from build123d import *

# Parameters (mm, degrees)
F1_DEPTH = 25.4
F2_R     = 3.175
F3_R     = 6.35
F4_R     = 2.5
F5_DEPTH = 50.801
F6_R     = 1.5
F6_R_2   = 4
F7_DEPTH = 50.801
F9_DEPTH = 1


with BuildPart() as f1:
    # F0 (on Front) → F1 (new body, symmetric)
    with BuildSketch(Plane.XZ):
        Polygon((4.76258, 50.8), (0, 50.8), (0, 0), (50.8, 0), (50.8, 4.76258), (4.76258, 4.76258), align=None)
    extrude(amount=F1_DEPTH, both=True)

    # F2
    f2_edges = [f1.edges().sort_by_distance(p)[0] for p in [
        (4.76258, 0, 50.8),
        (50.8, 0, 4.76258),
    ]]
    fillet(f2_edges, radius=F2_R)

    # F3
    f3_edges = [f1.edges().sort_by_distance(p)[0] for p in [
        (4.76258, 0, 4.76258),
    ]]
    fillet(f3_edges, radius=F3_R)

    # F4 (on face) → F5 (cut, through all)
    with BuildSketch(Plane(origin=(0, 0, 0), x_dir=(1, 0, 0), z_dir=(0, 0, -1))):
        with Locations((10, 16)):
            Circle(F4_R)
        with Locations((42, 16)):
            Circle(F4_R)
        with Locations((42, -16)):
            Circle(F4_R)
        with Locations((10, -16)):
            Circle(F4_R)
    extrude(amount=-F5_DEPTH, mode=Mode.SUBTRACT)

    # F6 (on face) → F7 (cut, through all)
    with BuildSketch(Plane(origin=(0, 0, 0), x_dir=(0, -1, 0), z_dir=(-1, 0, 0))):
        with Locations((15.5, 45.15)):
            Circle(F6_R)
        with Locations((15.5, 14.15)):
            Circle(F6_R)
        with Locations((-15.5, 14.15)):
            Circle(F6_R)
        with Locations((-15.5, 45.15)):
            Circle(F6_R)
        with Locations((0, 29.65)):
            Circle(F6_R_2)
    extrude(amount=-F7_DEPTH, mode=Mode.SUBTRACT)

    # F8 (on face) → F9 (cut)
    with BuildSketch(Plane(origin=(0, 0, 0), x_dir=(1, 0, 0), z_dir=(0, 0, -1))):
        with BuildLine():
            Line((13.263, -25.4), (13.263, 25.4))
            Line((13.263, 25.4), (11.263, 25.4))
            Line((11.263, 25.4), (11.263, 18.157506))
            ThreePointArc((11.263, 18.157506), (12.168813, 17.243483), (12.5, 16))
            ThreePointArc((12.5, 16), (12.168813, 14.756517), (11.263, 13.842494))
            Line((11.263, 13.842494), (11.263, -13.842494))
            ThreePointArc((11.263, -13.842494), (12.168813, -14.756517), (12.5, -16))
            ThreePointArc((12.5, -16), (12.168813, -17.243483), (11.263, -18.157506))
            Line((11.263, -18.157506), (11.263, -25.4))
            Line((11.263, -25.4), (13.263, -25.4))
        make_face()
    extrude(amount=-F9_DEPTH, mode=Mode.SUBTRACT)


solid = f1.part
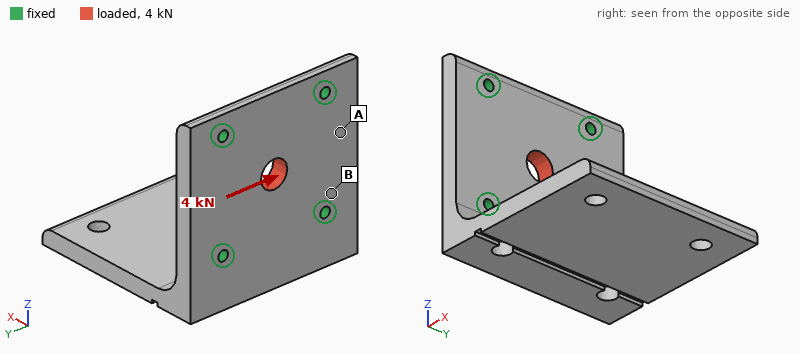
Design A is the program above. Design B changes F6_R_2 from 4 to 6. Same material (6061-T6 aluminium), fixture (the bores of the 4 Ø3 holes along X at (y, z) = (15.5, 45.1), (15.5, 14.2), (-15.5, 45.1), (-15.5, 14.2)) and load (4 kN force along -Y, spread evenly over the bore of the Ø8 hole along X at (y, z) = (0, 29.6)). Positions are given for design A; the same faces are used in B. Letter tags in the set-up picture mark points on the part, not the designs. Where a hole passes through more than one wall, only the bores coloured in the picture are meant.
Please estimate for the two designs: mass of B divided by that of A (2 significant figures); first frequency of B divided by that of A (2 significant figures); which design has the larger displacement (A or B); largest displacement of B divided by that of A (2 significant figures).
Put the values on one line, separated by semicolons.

0.99; 1.00; A; 0.85
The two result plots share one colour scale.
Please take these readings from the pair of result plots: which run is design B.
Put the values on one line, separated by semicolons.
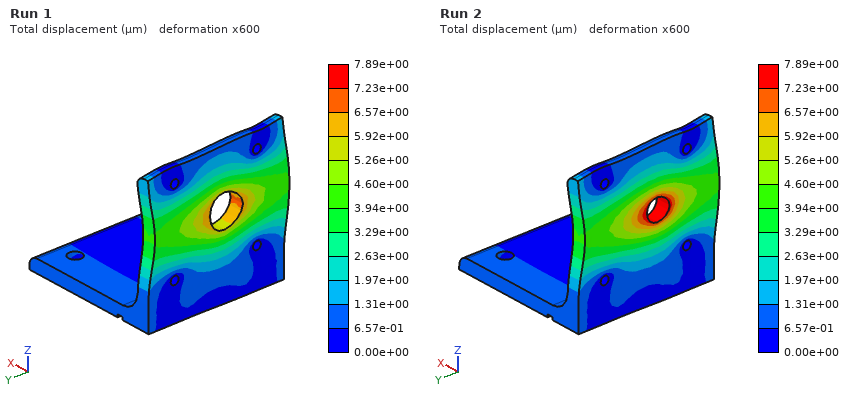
Run 1
